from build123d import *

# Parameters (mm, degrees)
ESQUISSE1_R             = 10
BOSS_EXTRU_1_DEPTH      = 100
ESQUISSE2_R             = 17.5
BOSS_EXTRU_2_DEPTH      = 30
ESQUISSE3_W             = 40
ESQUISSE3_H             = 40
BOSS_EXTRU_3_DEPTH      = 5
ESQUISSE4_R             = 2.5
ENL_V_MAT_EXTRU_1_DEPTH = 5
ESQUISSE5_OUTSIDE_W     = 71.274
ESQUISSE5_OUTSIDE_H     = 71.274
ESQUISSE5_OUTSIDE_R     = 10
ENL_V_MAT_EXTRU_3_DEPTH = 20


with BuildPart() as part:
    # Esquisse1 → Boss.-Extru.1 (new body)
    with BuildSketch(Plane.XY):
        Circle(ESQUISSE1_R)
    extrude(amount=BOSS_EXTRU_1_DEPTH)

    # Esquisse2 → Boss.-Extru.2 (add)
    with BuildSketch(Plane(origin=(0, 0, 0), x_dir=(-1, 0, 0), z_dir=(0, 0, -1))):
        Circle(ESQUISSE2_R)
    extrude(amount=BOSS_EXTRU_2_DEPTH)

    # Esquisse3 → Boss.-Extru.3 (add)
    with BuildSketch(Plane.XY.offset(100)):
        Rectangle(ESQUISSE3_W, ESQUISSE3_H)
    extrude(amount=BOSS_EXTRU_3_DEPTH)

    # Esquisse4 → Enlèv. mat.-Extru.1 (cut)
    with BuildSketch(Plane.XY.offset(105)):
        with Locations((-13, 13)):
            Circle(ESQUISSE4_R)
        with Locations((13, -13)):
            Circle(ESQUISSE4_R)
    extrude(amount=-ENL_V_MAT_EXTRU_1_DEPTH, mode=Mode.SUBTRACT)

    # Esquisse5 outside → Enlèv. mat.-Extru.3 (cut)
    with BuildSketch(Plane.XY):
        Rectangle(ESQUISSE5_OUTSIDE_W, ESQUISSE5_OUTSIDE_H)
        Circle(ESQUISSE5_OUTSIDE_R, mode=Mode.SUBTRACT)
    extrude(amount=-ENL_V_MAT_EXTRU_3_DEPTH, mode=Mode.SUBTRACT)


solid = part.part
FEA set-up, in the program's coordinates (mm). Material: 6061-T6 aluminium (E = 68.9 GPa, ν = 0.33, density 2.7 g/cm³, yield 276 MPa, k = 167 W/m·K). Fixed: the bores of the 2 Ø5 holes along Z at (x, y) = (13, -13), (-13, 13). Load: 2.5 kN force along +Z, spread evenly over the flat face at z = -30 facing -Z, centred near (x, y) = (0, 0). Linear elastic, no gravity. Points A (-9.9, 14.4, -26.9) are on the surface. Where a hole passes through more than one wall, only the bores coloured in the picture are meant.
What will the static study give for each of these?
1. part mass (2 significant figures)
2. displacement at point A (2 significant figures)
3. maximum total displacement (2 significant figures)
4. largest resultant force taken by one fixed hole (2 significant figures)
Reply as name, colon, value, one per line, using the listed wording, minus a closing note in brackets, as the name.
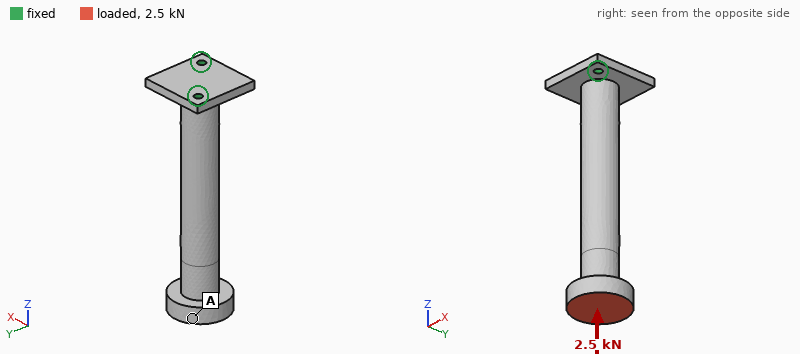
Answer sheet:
part mass: 150 g
displacement at point A: 31 µm
maximum total displacement: 31 µm
largest resultant force taken by one fixed hole: 1.3 kN
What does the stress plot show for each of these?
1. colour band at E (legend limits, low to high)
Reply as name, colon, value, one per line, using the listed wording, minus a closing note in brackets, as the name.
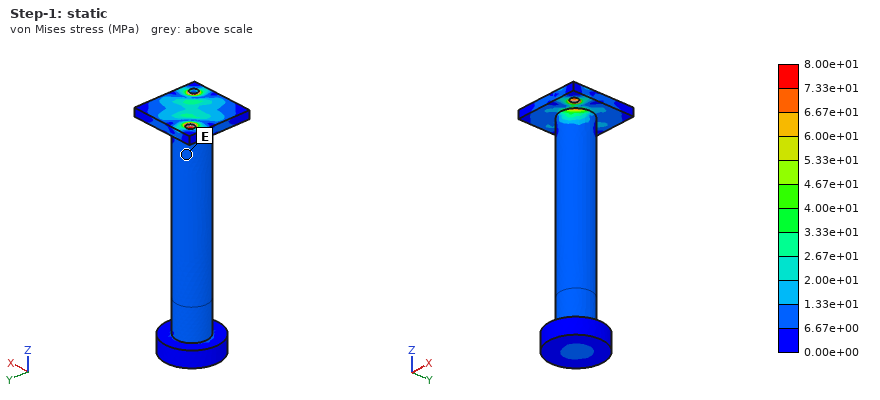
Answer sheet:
colour band at E: 6.67e+00 to 1.33e+01 MPa
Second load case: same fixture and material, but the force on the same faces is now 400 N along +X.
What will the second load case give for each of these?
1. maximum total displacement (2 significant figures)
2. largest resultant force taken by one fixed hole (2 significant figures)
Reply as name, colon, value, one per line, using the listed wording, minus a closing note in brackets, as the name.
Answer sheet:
maximum total displacement: 1.4 mm
largest resultant force taken by one fixed hole: 1.3 kN
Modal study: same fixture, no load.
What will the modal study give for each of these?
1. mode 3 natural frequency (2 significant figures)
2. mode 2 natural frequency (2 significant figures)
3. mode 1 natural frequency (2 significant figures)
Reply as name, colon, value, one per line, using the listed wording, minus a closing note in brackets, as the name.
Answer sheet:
mode 3 natural frequency: 3100 Hz
mode 2 natural frequency: 540 Hz
mode 1 natural frequency: 330 Hz
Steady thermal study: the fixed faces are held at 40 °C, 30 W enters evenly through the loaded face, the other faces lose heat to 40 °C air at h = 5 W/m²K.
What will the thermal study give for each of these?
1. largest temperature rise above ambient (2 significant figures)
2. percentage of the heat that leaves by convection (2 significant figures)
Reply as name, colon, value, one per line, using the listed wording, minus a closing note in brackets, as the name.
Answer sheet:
largest temperature rise above ambient: 78 K
percentage of the heat that leaves by convection: 7.8 %
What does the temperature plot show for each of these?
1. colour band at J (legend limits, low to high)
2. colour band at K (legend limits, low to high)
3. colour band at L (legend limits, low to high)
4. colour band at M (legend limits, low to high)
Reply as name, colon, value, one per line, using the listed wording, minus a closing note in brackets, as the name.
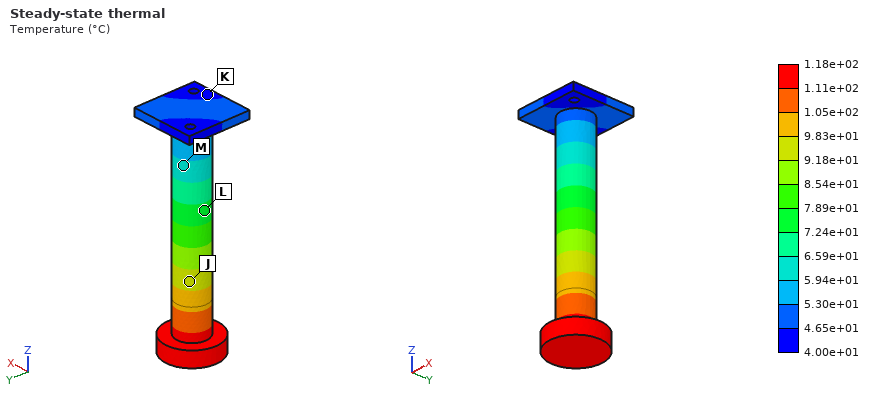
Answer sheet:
colour band at J: 9.18e+01 to 9.83e+01 °C
colour band at K: 4.00e+01 to 4.65e+01 °C
colour band at L: 7.24e+01 to 7.89e+01 °C
colour band at M: 5.94e+01 to 6.59e+01 °C
